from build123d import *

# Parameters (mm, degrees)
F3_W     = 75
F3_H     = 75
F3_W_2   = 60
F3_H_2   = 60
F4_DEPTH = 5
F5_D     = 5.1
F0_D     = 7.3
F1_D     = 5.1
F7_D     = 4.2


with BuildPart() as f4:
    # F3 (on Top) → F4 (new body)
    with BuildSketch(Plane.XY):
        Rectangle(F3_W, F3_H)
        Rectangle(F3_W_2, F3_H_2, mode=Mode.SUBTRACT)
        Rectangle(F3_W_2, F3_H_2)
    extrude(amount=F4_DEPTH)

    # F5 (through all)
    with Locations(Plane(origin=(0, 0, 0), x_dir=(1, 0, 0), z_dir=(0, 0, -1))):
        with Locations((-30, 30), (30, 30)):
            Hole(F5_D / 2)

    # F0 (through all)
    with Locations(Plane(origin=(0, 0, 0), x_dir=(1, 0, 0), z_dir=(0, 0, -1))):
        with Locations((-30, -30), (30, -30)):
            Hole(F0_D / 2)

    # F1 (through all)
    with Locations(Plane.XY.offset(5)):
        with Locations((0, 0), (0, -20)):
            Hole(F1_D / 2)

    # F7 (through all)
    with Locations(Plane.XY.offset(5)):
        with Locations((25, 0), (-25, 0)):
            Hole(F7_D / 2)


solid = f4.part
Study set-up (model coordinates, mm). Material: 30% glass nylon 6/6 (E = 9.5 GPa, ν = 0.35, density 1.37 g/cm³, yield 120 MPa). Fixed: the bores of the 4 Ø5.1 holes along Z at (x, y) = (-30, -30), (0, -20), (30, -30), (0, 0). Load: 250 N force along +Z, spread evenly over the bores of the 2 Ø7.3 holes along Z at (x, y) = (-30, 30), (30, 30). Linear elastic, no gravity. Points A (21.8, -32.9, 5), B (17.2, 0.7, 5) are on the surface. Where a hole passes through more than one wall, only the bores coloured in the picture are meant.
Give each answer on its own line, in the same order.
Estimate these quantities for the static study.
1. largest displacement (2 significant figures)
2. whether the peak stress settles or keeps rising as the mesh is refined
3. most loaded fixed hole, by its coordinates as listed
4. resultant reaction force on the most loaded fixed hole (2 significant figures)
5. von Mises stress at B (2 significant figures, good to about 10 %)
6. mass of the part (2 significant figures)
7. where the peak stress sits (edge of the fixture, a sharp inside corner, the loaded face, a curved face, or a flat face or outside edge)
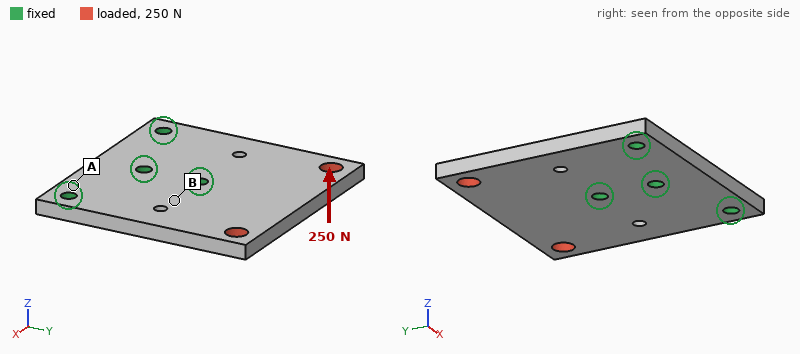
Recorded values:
0.81 mm
keeps rising
(0, 0)
400 N
16 MPa
37 g
edge of the fixture
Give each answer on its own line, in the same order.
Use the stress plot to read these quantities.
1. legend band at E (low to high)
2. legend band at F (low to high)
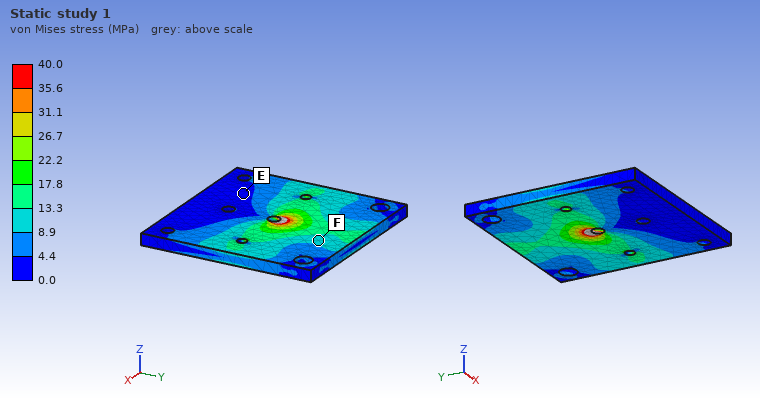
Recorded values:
0.0 to 4.4 MPa
8.9 to 13.3 MPa
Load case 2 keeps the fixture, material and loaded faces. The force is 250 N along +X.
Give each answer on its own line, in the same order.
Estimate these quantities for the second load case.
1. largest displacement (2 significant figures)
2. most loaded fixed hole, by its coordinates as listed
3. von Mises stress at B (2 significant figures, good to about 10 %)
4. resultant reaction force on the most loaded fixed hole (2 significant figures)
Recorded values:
20 µm
(0, 0)
1.2 MPa
260 N
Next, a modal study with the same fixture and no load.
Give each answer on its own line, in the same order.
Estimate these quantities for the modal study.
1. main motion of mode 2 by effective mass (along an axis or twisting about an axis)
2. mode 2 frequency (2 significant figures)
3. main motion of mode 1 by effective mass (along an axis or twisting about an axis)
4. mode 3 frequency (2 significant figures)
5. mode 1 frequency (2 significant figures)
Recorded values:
twisting about Y
1300 Hz
along Z
2900 Hz
1200 Hz
